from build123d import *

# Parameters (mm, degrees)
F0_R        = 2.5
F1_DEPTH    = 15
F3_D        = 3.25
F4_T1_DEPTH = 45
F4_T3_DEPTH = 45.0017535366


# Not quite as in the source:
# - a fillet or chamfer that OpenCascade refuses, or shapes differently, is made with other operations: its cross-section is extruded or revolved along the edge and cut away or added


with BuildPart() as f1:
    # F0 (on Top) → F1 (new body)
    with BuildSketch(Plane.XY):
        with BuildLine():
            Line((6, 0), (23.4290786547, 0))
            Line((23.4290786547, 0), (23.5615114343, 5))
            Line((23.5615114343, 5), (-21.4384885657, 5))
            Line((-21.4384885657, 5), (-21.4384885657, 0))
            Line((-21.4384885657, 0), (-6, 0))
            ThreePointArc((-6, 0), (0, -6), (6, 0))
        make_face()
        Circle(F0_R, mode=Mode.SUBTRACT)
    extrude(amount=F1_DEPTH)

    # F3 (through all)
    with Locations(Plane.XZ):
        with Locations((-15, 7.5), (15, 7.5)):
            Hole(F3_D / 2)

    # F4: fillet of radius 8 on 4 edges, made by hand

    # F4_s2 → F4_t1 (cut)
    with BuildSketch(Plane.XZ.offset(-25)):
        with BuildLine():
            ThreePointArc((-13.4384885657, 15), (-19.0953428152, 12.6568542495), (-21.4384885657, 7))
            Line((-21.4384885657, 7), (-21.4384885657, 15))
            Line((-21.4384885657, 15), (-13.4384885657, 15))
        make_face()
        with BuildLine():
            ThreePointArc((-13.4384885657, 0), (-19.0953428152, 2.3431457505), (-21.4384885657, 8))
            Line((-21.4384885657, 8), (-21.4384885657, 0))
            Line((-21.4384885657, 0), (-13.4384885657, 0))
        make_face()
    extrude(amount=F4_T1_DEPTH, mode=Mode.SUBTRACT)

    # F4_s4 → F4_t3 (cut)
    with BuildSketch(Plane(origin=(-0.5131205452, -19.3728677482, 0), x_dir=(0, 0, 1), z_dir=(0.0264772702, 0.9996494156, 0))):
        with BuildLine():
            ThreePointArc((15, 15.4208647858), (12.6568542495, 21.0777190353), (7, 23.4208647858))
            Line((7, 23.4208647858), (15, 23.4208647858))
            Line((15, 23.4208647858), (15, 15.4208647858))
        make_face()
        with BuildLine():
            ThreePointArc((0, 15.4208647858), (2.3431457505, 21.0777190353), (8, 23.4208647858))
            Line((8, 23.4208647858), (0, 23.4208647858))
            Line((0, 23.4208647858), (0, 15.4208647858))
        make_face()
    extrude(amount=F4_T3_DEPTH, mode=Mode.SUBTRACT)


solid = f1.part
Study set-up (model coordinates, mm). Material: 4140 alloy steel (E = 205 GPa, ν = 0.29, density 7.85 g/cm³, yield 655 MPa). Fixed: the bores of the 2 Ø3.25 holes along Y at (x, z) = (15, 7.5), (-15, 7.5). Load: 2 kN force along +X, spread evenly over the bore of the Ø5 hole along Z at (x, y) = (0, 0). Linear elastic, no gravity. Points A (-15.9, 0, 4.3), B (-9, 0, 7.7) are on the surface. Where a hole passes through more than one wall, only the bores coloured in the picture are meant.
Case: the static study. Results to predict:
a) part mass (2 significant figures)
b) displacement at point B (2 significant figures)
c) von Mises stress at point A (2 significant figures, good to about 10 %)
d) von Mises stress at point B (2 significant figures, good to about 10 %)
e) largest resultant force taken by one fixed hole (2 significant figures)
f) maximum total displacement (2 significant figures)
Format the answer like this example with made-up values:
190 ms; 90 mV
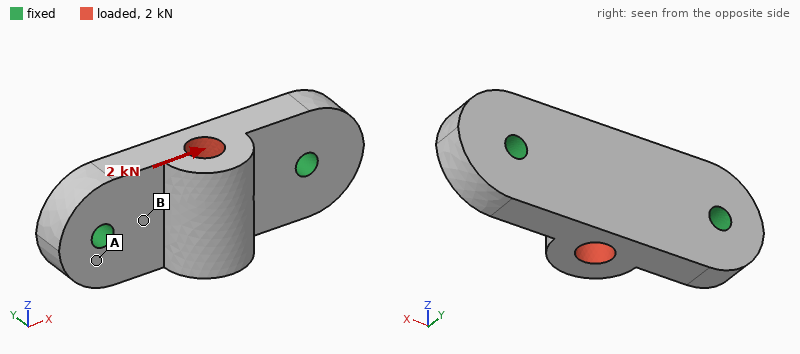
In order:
28 g; 0.59 µm; 6.9 MPa; 29 MPa; 1.0 kN; 2.0 µm
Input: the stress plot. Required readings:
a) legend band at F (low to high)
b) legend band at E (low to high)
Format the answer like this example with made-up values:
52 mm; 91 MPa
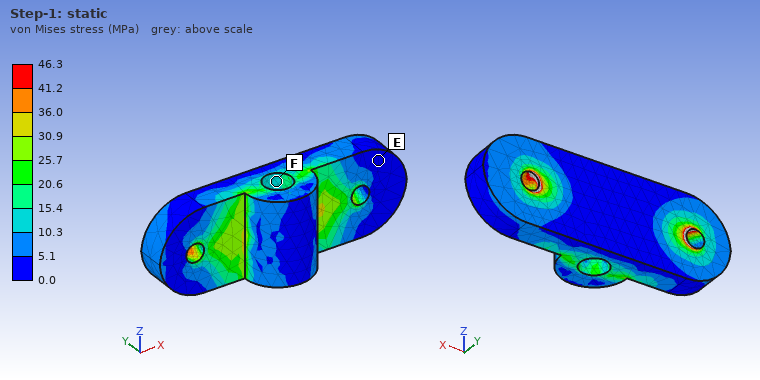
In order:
10.3 to 15.4 MPa; 0.0 to 5.1 MPa
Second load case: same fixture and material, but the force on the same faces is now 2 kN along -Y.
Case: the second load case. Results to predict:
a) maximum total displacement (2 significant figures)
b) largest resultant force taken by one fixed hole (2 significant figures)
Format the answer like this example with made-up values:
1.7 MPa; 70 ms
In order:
8.7 µm; 1.0 kN
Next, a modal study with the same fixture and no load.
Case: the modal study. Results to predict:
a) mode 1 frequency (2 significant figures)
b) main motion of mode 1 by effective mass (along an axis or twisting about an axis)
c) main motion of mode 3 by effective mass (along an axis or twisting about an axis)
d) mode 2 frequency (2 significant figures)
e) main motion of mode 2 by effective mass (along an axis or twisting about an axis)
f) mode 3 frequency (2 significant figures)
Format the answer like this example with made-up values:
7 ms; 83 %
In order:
20 kHz; along Z; along Z; 22 kHz; along Y; 31 kHz
